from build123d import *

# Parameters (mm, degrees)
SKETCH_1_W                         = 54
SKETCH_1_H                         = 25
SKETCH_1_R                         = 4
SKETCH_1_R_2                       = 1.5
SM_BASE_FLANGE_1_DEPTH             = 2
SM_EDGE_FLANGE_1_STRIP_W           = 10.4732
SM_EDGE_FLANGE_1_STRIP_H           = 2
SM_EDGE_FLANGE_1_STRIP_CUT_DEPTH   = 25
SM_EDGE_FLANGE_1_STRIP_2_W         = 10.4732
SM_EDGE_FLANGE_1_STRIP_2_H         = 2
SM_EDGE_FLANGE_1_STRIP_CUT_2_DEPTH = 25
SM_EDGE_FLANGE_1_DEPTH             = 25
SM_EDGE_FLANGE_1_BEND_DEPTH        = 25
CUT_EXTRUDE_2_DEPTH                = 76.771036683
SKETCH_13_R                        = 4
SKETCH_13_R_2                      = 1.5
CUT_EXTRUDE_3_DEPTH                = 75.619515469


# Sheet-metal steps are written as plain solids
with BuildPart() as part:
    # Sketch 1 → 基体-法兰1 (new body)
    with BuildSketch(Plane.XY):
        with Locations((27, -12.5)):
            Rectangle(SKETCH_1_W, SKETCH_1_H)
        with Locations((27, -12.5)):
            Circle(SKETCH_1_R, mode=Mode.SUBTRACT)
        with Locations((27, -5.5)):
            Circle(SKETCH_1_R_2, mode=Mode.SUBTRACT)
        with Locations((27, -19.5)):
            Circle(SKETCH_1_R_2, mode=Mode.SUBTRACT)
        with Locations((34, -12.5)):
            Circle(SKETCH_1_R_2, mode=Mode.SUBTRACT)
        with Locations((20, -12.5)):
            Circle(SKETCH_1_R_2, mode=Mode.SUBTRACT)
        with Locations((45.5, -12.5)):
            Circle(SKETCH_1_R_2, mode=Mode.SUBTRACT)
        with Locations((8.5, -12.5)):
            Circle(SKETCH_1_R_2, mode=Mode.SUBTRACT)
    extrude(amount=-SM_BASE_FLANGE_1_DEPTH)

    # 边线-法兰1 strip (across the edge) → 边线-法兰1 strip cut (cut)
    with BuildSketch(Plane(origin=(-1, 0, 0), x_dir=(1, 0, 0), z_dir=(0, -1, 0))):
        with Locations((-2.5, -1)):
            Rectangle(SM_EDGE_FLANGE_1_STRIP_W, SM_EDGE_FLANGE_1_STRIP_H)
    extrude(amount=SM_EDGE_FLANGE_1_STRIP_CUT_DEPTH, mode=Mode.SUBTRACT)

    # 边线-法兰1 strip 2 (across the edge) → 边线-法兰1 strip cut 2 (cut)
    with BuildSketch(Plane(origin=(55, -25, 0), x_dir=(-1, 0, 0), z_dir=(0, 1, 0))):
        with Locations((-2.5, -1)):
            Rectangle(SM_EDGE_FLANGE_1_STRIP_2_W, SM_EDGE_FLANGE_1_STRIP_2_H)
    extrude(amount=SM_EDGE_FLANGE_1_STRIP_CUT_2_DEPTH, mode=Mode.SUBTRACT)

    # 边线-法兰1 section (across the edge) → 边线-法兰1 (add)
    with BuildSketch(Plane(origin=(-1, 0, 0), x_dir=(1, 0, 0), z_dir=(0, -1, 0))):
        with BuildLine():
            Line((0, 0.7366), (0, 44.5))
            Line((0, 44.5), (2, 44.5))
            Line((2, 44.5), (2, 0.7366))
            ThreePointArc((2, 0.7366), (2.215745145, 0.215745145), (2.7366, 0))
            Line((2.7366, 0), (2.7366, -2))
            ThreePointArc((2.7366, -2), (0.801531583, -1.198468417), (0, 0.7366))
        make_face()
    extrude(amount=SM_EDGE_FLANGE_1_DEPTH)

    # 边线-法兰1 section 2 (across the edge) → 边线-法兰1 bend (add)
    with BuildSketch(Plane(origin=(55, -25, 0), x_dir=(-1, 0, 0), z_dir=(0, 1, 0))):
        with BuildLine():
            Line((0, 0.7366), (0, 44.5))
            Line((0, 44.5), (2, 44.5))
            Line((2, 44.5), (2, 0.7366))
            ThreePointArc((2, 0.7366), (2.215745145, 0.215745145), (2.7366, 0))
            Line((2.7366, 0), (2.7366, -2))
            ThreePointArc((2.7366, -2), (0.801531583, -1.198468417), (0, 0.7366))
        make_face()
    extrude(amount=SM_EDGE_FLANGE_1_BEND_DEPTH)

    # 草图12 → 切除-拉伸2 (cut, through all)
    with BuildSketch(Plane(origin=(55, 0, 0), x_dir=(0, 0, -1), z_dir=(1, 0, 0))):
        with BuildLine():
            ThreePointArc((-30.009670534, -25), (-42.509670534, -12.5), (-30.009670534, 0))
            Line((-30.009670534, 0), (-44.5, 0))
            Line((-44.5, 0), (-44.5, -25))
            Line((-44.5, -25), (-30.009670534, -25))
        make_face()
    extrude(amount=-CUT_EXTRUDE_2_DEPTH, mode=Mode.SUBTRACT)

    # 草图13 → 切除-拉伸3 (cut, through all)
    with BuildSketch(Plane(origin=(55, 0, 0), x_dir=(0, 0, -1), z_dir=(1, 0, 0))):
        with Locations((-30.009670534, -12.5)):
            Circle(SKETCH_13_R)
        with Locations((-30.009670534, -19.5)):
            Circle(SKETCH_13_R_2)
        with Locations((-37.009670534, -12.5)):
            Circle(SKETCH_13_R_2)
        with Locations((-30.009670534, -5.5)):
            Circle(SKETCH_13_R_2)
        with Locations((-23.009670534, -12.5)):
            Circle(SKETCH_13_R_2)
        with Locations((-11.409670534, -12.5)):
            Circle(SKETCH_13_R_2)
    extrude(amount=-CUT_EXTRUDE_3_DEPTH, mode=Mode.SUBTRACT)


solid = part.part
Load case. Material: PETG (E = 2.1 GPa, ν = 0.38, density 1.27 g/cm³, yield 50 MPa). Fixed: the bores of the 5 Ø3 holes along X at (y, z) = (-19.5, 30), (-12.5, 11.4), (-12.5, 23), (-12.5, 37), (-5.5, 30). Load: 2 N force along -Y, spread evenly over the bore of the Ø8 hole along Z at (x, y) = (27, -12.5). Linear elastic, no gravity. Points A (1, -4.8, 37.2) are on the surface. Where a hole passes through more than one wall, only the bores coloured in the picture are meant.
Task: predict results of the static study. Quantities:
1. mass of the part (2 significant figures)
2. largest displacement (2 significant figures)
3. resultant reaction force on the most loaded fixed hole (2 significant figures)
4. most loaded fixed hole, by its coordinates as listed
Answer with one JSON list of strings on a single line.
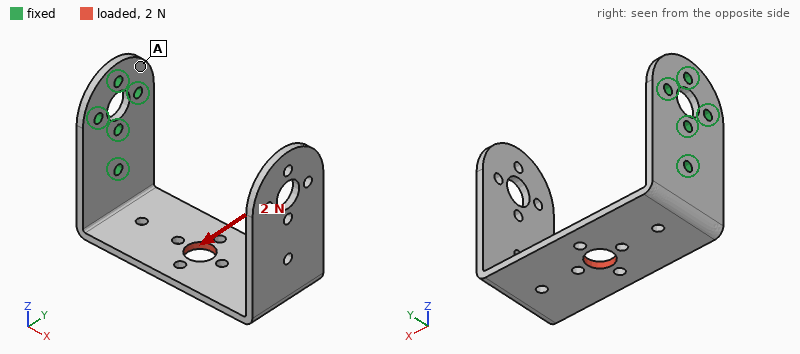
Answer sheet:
["7.8 g", "0.76 mm", "2.8 N", "(-12.5, 11.4)"]
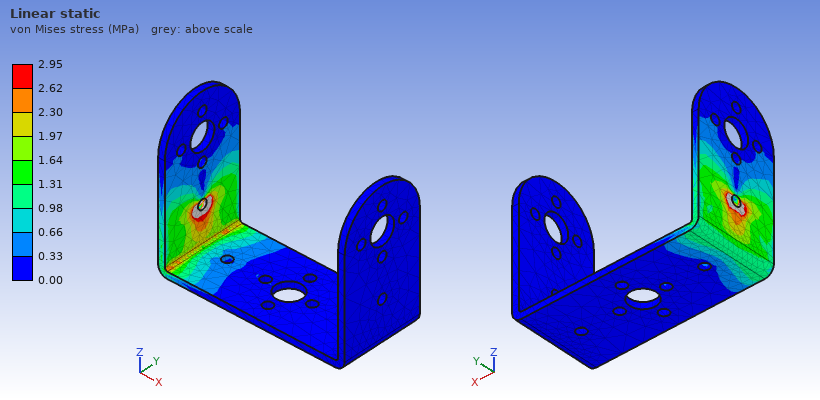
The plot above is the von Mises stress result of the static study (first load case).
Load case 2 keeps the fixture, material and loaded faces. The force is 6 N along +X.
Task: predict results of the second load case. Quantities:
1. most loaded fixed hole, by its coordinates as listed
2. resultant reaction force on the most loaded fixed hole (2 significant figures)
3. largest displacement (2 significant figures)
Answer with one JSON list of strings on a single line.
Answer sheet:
["(-12.5, 11.4)", "8.3 N", "0.86 mm"]
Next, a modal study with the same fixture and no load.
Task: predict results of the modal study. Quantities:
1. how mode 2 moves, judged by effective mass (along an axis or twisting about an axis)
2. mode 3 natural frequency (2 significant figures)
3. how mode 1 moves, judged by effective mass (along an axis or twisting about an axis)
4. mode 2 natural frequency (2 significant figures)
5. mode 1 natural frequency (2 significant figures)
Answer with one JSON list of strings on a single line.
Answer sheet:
["along Y", "170 Hz", "along Z", "85 Hz", "50 Hz"]
